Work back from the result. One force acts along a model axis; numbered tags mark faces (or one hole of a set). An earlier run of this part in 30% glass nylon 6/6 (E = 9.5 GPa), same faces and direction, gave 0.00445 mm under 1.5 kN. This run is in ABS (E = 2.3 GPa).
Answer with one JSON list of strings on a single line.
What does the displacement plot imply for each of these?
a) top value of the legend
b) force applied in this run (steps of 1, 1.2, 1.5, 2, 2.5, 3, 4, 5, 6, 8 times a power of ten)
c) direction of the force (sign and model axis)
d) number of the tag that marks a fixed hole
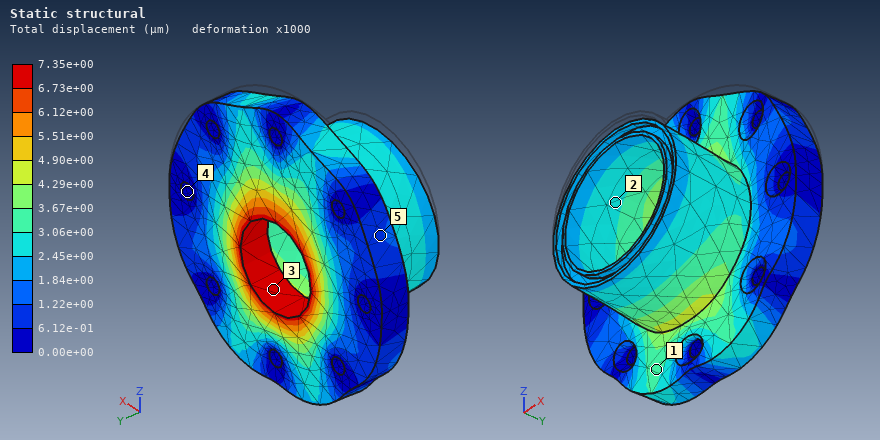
["7.35e+00 µm", "600 N", "-Z", "4"]
